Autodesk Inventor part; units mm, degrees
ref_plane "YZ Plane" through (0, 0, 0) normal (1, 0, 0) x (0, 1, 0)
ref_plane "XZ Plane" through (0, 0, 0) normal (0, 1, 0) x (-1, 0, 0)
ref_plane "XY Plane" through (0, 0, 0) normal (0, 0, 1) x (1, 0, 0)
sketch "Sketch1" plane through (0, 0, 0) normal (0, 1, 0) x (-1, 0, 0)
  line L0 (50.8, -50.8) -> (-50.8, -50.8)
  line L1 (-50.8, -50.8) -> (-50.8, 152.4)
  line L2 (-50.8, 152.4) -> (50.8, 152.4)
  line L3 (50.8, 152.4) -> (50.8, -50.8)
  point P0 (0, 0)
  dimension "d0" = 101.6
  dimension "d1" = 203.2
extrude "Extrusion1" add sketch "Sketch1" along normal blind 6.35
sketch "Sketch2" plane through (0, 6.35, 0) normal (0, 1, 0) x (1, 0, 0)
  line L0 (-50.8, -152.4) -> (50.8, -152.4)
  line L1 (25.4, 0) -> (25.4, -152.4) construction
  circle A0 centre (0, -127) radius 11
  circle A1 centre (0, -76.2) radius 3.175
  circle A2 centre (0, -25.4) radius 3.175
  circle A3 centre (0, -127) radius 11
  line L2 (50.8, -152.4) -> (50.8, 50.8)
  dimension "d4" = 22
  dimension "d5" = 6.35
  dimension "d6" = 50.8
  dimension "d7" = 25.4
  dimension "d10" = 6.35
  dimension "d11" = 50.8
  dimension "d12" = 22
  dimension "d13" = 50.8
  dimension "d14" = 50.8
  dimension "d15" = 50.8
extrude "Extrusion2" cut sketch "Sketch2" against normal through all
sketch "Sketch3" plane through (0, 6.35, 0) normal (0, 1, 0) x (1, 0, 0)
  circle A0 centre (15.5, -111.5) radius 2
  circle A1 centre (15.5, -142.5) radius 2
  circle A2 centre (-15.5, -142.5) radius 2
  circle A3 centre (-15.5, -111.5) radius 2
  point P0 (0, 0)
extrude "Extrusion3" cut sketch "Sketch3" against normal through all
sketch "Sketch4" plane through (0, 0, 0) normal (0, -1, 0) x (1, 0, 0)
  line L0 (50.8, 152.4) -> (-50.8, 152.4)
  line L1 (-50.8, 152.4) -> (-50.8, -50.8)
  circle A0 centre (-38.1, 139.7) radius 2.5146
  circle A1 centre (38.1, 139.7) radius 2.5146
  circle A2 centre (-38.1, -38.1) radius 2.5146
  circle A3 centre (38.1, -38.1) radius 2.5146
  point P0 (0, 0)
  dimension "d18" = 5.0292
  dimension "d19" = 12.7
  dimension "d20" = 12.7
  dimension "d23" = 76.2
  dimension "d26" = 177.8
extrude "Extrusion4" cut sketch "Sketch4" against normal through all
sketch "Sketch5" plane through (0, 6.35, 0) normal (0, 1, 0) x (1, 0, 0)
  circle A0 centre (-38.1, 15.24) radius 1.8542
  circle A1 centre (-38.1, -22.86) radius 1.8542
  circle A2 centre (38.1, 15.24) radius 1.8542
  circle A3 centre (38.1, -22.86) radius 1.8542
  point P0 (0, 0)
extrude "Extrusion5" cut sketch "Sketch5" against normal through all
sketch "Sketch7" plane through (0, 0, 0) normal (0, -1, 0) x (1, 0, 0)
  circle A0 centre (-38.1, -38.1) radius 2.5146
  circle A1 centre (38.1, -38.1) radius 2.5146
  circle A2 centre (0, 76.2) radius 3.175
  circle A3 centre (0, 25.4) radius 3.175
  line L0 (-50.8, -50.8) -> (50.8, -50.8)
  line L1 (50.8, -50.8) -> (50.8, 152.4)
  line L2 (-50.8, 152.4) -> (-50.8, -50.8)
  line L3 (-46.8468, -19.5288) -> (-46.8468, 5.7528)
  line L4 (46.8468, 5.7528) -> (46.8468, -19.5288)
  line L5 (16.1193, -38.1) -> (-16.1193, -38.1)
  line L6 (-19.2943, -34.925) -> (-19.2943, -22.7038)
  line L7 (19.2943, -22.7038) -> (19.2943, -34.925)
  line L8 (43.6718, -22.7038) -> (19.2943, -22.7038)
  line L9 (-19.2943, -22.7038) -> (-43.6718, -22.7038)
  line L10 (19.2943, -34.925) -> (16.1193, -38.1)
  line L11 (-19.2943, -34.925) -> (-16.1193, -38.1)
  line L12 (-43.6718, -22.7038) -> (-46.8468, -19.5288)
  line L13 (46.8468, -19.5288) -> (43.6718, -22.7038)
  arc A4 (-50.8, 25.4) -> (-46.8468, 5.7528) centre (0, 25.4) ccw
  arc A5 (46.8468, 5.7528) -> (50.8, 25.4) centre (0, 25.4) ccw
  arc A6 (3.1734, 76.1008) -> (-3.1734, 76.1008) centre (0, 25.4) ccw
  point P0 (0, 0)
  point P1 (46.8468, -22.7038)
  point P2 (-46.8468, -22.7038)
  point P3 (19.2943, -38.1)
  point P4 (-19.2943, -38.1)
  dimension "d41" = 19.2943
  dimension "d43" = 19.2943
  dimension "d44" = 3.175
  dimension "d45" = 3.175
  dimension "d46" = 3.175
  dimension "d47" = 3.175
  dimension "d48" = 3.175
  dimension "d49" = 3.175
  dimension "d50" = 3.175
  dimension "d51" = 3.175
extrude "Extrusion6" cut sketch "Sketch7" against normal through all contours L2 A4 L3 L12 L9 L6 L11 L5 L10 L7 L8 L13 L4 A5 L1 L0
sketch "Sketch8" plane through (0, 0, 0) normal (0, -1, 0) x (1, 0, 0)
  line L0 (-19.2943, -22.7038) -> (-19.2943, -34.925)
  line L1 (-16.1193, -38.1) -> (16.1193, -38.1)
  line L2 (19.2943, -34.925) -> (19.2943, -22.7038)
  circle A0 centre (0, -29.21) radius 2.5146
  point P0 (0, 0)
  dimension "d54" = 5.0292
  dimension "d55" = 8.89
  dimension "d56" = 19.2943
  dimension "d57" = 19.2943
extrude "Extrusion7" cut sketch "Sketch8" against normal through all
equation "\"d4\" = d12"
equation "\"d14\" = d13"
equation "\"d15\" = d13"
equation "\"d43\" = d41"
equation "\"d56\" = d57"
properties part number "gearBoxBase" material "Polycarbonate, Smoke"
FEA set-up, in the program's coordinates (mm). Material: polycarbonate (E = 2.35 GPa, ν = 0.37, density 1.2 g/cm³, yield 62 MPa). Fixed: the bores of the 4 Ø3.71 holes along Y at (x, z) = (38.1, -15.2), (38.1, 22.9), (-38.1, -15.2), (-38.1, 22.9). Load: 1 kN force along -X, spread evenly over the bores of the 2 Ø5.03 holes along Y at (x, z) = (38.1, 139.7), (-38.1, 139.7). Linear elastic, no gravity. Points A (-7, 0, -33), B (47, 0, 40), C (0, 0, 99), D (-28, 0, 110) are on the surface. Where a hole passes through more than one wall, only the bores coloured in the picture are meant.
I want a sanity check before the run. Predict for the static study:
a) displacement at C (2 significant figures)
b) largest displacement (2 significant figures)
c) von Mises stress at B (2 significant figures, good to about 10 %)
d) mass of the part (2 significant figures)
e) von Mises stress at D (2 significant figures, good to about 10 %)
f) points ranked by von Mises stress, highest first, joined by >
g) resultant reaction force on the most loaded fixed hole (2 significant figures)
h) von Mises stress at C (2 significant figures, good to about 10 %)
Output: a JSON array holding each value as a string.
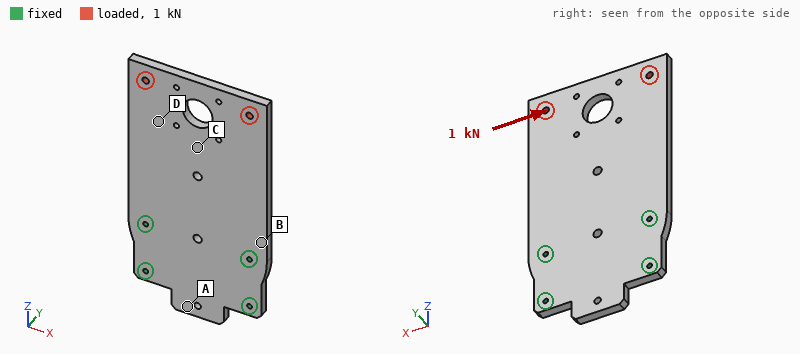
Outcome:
["0.45 mm", "0.97 mm", "7.9 MPa", "130 g", "3.2 MPa", "B > C > D > A", "1.4 kN", "5.8 MPa"]
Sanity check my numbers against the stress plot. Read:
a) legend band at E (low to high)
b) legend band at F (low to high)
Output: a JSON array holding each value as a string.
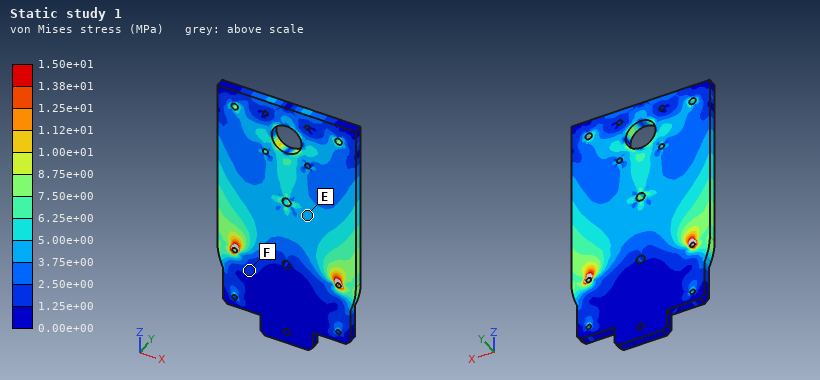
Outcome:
["3.75e+00 to 5.00e+00 MPa", "1.25e+00 to 2.50e+00 MPa"]
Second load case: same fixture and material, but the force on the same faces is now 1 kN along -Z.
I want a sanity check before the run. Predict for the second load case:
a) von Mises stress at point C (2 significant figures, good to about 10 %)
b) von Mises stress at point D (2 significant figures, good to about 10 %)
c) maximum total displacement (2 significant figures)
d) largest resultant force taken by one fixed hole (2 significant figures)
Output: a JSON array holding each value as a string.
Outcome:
["0.76 MPa", "1.8 MPa", "0.12 mm", "380 N"]
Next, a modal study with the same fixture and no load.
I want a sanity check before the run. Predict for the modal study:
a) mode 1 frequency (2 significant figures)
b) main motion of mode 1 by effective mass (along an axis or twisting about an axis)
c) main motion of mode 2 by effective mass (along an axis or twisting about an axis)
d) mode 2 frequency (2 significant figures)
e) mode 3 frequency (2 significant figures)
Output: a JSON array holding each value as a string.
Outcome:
["83 Hz", "along Y", "twisting about Z", "240 Hz", "490 Hz"]
